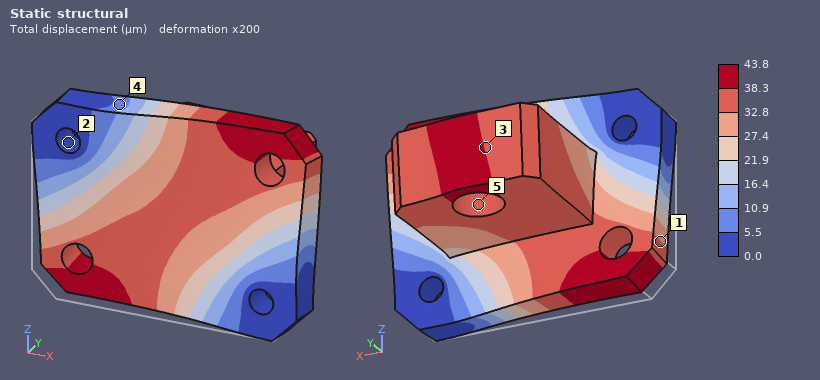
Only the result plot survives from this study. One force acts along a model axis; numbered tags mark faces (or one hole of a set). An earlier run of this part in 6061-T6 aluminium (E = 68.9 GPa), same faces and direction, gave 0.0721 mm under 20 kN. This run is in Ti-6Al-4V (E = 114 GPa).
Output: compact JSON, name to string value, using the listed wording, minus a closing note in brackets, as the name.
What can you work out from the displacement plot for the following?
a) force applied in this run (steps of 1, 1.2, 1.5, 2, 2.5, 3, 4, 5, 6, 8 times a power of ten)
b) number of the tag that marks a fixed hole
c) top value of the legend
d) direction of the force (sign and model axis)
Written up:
{"force applied in this run": "20 kN", "number of the tag that marks a fixed hole": "2", "top value of the legend": "43.8 µm", "direction of the force": "+Y"}
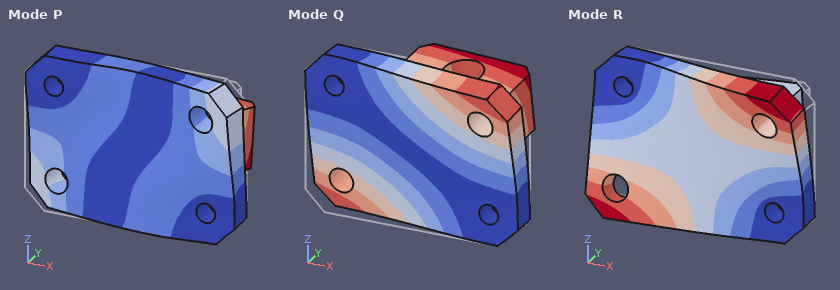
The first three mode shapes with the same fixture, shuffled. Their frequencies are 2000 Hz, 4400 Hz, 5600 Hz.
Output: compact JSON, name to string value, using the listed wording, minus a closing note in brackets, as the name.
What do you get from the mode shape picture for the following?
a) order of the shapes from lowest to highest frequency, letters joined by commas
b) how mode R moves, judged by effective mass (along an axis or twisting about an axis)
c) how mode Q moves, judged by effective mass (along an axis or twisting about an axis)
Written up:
{"order of the shapes from lowest to highest frequency, letters joined by commas": "Q, R, P", "how mode R moves, judged by effective mass": "along Y", "how mode Q moves, judged by effective mass": "along Z"}
